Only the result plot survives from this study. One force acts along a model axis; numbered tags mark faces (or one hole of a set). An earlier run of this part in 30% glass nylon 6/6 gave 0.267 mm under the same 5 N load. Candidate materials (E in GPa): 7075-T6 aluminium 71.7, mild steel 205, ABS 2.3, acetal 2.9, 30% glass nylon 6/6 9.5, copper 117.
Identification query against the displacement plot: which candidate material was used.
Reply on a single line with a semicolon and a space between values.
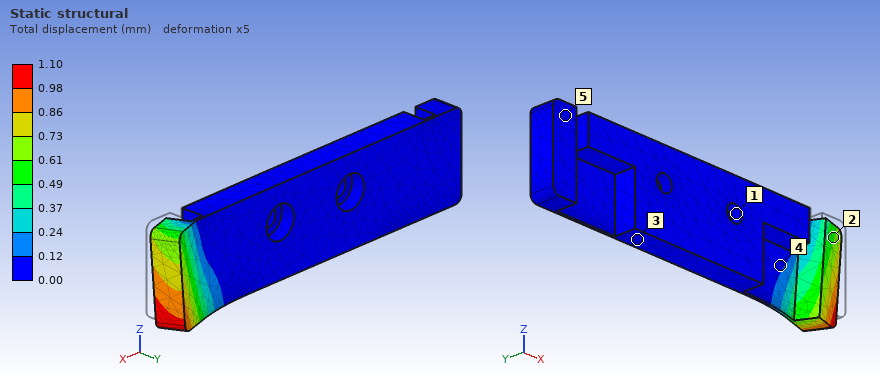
ABS
